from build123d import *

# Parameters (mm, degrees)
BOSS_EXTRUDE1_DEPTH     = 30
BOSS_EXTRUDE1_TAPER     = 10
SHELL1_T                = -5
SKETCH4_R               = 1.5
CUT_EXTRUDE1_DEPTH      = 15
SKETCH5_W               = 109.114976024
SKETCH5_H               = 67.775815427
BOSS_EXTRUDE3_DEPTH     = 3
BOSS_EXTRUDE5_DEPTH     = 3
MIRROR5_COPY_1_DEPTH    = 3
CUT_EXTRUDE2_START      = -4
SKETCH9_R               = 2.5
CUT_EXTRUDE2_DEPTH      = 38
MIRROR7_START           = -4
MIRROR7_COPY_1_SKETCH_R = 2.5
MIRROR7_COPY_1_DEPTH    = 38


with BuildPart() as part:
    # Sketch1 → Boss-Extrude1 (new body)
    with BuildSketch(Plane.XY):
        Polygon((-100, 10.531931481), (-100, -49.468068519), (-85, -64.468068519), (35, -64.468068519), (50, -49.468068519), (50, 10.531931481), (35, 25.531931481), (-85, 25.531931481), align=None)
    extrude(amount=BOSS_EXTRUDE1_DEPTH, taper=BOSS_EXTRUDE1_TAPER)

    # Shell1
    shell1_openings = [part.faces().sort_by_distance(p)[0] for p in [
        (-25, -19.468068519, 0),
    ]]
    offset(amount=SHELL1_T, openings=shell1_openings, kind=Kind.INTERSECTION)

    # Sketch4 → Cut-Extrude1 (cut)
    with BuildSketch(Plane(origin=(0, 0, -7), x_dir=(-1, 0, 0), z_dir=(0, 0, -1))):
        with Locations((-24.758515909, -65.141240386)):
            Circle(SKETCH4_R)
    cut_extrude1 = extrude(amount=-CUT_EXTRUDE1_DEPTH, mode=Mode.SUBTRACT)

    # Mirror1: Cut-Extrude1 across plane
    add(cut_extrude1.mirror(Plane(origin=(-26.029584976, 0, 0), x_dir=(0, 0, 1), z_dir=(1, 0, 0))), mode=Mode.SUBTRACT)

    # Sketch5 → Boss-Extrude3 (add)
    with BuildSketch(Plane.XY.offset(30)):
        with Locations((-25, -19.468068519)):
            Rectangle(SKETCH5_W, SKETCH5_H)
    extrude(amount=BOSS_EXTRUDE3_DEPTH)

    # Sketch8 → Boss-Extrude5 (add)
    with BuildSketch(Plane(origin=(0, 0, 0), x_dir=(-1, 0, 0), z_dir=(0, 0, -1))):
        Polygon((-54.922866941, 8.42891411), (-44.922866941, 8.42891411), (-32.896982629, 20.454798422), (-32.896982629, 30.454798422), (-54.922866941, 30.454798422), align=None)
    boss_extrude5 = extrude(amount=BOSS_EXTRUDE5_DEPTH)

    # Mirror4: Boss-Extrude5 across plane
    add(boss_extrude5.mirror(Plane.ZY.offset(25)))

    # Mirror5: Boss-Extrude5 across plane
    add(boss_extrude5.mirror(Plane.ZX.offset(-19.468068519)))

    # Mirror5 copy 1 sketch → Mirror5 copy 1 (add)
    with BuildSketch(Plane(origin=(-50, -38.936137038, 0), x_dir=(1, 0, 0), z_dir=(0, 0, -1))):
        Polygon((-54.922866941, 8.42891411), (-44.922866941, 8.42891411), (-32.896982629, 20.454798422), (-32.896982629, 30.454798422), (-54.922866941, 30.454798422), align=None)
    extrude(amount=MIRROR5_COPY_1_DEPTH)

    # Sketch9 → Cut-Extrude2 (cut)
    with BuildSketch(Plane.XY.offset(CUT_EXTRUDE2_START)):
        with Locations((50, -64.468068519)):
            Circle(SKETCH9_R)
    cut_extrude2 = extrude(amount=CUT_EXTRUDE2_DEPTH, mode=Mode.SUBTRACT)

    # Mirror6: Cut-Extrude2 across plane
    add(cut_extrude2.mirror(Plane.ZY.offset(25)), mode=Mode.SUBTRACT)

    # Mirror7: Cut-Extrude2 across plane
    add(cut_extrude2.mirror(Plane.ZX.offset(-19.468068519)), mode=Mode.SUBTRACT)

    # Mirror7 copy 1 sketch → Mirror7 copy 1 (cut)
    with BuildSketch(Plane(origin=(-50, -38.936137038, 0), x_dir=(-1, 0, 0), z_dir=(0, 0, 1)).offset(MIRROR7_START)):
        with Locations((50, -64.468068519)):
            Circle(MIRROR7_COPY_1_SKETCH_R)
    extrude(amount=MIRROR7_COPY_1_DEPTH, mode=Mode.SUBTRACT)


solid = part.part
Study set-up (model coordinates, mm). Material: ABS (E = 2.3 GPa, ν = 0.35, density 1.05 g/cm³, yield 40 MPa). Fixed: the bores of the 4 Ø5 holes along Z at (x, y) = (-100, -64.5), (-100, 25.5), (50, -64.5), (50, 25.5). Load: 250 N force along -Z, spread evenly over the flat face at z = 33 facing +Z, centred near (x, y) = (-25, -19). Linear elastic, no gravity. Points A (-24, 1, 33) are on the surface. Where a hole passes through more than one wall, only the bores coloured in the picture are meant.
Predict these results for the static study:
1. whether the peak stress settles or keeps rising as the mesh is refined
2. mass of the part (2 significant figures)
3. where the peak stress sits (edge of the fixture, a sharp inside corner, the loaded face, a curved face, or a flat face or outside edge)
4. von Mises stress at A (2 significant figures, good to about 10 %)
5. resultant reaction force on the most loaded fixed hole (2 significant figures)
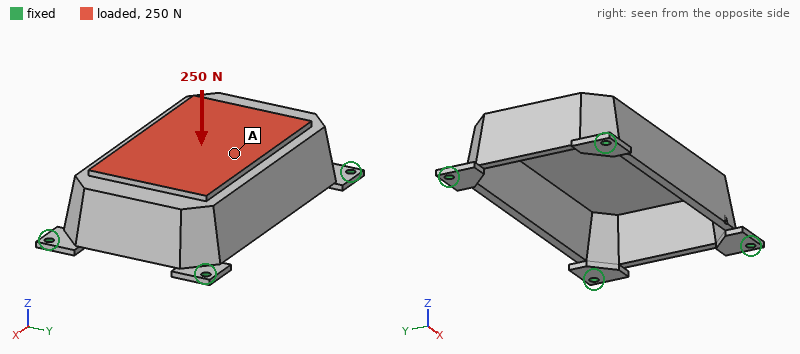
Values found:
keeps rising
140 g
edge of the fixture
0.98 MPa
91 N
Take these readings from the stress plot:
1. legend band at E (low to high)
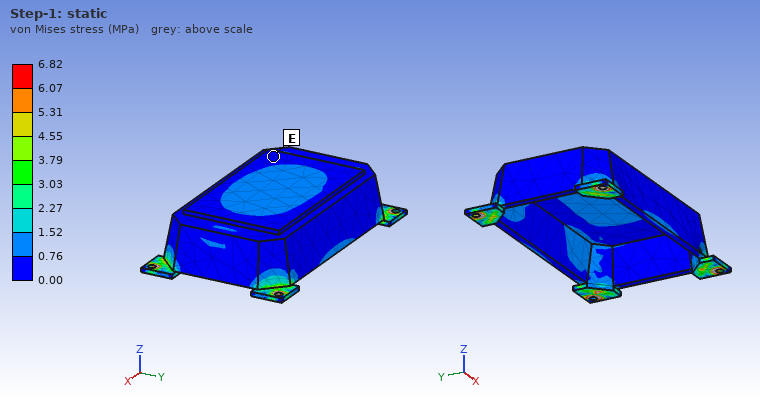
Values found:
0.00 to 0.76 MPa
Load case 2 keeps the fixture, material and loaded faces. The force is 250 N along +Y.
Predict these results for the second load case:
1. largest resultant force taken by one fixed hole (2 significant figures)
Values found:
85 N
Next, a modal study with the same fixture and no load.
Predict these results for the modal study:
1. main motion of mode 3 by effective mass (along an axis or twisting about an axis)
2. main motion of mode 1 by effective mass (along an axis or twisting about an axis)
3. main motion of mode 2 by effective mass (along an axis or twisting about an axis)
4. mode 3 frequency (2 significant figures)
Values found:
along Y
along Z
along Y
890 Hz
